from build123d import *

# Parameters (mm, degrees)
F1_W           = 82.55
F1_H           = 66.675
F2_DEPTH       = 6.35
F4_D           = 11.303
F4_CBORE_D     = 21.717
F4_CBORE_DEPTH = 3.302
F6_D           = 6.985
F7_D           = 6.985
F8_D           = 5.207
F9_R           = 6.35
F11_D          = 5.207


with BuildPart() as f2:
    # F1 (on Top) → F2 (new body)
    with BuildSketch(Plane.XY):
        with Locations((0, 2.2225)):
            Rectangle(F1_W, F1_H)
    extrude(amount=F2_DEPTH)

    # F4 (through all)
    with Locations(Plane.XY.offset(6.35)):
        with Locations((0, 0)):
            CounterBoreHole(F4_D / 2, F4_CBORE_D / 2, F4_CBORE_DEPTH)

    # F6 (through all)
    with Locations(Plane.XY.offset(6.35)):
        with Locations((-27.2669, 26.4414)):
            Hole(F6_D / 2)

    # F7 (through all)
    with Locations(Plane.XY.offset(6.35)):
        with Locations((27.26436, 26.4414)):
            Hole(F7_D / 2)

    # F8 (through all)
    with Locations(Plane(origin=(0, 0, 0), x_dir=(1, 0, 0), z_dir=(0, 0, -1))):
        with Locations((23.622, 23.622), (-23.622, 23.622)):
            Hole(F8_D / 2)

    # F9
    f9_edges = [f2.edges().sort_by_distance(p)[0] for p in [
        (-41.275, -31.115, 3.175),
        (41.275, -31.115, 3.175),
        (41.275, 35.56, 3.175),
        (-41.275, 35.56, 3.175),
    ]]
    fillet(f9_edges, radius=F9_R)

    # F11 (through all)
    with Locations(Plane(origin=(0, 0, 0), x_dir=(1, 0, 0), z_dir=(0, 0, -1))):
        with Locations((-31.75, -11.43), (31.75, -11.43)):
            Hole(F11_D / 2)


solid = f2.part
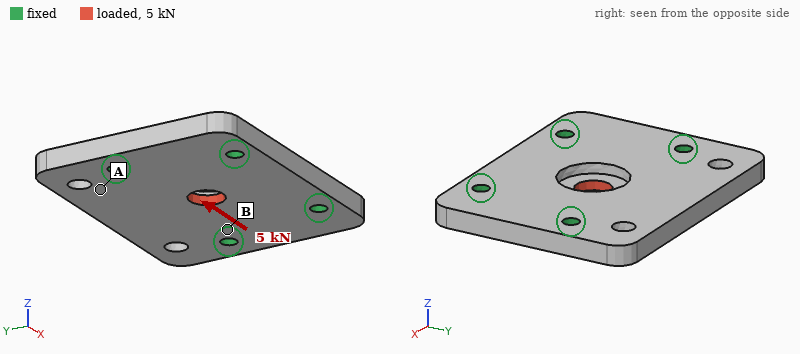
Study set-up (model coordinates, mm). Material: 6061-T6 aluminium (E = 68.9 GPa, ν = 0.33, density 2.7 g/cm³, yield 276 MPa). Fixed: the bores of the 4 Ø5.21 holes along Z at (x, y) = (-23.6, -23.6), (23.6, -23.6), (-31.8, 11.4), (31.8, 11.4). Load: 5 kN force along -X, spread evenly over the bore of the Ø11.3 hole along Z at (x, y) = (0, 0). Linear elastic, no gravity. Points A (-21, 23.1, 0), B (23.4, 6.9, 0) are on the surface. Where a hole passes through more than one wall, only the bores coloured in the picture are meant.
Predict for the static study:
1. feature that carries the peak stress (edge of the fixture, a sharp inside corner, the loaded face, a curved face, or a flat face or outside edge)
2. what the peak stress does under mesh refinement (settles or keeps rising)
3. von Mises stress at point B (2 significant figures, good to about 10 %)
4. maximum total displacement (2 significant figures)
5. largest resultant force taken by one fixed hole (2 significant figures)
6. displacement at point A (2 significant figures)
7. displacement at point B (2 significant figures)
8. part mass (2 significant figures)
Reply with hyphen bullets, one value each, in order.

- a sharp inside corner
- keeps rising
- 18 MPa
- 11 µm
- 1.5 kN
- 2.3 µm
- 2.0 µm
- 87 g
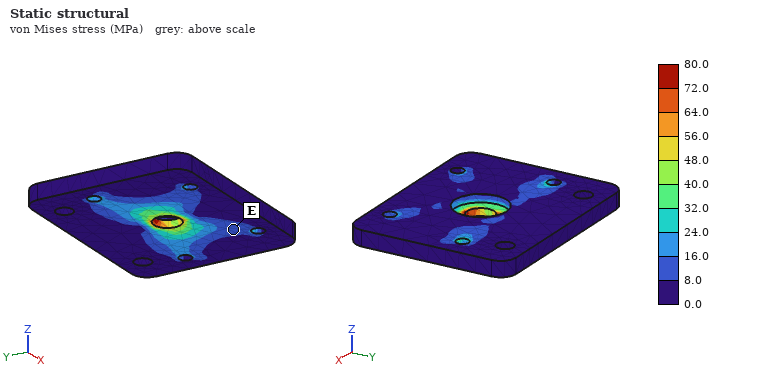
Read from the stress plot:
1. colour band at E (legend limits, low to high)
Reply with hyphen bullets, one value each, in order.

- 8.0 to 16.0 MPa
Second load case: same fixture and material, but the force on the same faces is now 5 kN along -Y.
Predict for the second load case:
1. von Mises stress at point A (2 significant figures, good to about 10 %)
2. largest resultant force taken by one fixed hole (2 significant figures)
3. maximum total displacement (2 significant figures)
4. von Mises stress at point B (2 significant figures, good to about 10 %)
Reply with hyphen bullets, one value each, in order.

- 8.7 MPa
- 1.6 kN
- 14 µm
- 13 MPa
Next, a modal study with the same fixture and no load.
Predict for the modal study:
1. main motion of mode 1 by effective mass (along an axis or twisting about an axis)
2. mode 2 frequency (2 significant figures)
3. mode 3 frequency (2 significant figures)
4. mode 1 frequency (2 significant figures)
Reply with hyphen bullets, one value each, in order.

- along Z
- 10 kHz
- 10 kHz
- 5500 Hz
